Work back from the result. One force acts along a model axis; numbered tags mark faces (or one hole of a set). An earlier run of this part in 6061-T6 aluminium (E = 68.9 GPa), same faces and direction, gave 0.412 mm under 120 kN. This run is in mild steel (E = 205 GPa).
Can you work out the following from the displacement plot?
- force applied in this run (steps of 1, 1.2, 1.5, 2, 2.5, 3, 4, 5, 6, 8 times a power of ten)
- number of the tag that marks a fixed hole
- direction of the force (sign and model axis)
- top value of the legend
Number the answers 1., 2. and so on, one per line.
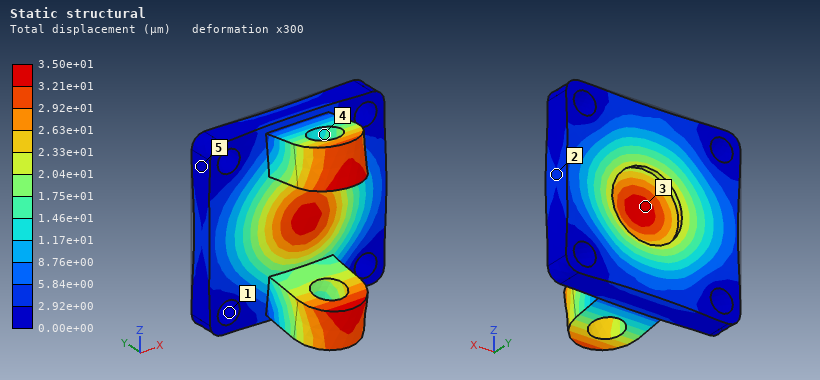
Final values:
1. 30 kN
2. 1
3. -Y
4. 3.50e+01 µm
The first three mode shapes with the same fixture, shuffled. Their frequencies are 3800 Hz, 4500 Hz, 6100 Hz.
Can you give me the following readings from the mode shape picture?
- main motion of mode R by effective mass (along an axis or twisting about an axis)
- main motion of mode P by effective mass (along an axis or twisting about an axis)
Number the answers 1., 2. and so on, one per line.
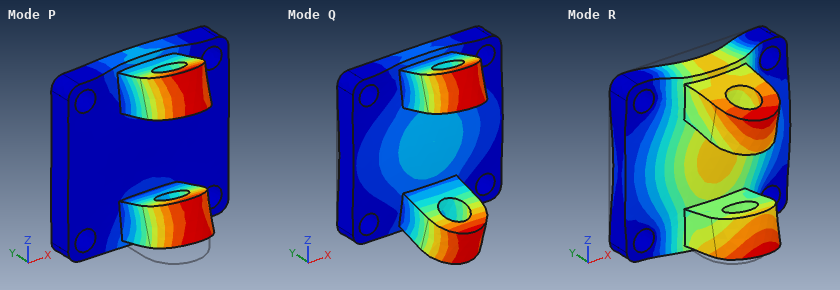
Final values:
1. along Y
2. along Z
